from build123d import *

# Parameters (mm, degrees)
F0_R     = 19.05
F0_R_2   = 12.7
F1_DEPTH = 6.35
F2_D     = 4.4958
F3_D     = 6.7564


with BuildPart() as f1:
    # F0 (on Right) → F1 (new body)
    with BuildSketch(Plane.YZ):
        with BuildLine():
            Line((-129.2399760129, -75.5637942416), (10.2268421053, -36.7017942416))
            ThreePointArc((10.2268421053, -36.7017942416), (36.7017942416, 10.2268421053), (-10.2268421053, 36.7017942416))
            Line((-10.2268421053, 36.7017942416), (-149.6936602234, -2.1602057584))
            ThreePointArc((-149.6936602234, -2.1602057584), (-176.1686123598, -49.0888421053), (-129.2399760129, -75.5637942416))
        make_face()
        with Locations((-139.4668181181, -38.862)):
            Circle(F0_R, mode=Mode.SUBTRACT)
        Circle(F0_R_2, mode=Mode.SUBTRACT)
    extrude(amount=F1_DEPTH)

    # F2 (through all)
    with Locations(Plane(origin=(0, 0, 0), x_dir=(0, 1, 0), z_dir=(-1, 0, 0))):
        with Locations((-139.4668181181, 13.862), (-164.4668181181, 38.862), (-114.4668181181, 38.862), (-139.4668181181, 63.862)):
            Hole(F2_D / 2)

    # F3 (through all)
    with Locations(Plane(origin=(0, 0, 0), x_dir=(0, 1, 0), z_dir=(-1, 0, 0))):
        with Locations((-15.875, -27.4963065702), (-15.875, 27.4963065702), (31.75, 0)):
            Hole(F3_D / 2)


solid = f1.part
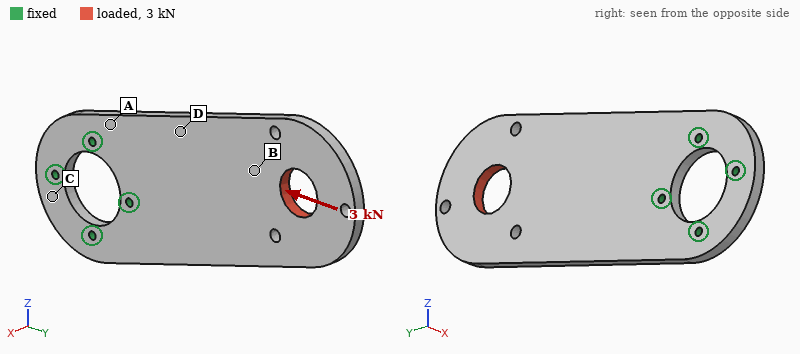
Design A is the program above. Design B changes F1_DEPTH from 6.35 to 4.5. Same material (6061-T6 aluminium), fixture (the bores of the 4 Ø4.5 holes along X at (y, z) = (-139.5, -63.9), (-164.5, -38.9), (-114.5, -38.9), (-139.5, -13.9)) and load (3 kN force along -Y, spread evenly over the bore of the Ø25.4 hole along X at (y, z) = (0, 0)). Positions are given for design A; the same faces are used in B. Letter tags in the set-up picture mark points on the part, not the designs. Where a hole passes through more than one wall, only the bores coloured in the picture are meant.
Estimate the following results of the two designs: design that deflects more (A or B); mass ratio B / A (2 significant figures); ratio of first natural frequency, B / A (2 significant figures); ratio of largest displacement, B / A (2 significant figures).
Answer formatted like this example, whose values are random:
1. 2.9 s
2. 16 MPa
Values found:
1. B
2. 0.71
3. 0.72
4. 1.4
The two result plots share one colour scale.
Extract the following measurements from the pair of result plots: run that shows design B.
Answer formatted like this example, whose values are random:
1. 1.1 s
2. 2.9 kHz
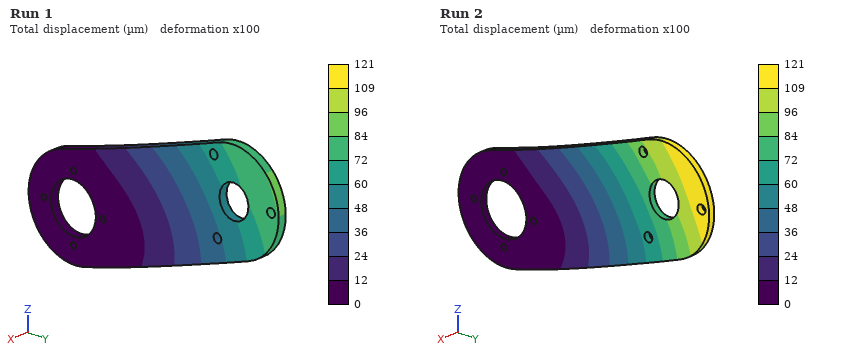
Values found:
1. Run 2
